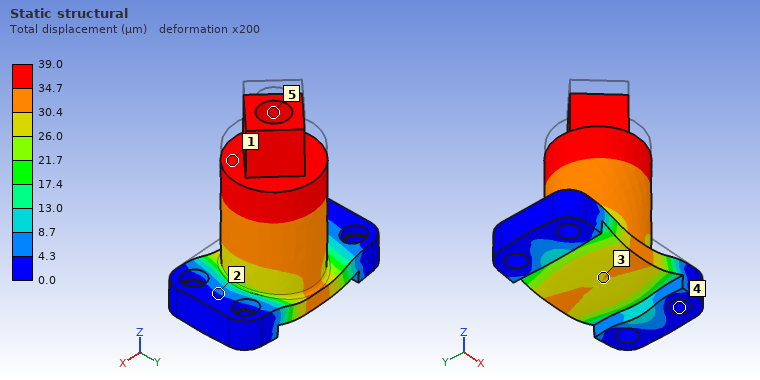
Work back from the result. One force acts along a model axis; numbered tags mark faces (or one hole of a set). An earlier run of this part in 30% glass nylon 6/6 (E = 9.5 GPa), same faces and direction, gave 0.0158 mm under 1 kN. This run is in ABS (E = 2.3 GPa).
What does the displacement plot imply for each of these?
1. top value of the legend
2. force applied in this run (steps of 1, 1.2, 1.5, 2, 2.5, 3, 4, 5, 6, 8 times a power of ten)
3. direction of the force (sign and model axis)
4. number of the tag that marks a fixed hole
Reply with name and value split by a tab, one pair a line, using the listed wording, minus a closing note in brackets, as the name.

top value of the legend	39.0 µm
force applied in this run	600 N
direction of the force	-Z
number of the tag that marks a fixed hole	4
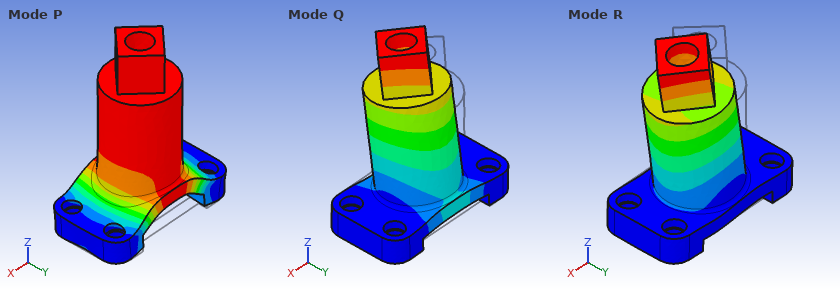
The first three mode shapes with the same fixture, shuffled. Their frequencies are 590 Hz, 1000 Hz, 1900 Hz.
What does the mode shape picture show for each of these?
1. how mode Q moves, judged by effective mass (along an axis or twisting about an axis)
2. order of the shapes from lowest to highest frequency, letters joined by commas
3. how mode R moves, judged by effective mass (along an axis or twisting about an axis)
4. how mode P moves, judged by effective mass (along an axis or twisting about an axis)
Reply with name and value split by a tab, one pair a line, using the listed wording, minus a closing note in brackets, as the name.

how mode Q moves, judged by effective mass	along Y
order of the shapes from lowest to highest frequency, letters joined by commas	Q, R, P
how mode R moves, judged by effective mass	along X
how mode P moves, judged by effective mass	along Z
